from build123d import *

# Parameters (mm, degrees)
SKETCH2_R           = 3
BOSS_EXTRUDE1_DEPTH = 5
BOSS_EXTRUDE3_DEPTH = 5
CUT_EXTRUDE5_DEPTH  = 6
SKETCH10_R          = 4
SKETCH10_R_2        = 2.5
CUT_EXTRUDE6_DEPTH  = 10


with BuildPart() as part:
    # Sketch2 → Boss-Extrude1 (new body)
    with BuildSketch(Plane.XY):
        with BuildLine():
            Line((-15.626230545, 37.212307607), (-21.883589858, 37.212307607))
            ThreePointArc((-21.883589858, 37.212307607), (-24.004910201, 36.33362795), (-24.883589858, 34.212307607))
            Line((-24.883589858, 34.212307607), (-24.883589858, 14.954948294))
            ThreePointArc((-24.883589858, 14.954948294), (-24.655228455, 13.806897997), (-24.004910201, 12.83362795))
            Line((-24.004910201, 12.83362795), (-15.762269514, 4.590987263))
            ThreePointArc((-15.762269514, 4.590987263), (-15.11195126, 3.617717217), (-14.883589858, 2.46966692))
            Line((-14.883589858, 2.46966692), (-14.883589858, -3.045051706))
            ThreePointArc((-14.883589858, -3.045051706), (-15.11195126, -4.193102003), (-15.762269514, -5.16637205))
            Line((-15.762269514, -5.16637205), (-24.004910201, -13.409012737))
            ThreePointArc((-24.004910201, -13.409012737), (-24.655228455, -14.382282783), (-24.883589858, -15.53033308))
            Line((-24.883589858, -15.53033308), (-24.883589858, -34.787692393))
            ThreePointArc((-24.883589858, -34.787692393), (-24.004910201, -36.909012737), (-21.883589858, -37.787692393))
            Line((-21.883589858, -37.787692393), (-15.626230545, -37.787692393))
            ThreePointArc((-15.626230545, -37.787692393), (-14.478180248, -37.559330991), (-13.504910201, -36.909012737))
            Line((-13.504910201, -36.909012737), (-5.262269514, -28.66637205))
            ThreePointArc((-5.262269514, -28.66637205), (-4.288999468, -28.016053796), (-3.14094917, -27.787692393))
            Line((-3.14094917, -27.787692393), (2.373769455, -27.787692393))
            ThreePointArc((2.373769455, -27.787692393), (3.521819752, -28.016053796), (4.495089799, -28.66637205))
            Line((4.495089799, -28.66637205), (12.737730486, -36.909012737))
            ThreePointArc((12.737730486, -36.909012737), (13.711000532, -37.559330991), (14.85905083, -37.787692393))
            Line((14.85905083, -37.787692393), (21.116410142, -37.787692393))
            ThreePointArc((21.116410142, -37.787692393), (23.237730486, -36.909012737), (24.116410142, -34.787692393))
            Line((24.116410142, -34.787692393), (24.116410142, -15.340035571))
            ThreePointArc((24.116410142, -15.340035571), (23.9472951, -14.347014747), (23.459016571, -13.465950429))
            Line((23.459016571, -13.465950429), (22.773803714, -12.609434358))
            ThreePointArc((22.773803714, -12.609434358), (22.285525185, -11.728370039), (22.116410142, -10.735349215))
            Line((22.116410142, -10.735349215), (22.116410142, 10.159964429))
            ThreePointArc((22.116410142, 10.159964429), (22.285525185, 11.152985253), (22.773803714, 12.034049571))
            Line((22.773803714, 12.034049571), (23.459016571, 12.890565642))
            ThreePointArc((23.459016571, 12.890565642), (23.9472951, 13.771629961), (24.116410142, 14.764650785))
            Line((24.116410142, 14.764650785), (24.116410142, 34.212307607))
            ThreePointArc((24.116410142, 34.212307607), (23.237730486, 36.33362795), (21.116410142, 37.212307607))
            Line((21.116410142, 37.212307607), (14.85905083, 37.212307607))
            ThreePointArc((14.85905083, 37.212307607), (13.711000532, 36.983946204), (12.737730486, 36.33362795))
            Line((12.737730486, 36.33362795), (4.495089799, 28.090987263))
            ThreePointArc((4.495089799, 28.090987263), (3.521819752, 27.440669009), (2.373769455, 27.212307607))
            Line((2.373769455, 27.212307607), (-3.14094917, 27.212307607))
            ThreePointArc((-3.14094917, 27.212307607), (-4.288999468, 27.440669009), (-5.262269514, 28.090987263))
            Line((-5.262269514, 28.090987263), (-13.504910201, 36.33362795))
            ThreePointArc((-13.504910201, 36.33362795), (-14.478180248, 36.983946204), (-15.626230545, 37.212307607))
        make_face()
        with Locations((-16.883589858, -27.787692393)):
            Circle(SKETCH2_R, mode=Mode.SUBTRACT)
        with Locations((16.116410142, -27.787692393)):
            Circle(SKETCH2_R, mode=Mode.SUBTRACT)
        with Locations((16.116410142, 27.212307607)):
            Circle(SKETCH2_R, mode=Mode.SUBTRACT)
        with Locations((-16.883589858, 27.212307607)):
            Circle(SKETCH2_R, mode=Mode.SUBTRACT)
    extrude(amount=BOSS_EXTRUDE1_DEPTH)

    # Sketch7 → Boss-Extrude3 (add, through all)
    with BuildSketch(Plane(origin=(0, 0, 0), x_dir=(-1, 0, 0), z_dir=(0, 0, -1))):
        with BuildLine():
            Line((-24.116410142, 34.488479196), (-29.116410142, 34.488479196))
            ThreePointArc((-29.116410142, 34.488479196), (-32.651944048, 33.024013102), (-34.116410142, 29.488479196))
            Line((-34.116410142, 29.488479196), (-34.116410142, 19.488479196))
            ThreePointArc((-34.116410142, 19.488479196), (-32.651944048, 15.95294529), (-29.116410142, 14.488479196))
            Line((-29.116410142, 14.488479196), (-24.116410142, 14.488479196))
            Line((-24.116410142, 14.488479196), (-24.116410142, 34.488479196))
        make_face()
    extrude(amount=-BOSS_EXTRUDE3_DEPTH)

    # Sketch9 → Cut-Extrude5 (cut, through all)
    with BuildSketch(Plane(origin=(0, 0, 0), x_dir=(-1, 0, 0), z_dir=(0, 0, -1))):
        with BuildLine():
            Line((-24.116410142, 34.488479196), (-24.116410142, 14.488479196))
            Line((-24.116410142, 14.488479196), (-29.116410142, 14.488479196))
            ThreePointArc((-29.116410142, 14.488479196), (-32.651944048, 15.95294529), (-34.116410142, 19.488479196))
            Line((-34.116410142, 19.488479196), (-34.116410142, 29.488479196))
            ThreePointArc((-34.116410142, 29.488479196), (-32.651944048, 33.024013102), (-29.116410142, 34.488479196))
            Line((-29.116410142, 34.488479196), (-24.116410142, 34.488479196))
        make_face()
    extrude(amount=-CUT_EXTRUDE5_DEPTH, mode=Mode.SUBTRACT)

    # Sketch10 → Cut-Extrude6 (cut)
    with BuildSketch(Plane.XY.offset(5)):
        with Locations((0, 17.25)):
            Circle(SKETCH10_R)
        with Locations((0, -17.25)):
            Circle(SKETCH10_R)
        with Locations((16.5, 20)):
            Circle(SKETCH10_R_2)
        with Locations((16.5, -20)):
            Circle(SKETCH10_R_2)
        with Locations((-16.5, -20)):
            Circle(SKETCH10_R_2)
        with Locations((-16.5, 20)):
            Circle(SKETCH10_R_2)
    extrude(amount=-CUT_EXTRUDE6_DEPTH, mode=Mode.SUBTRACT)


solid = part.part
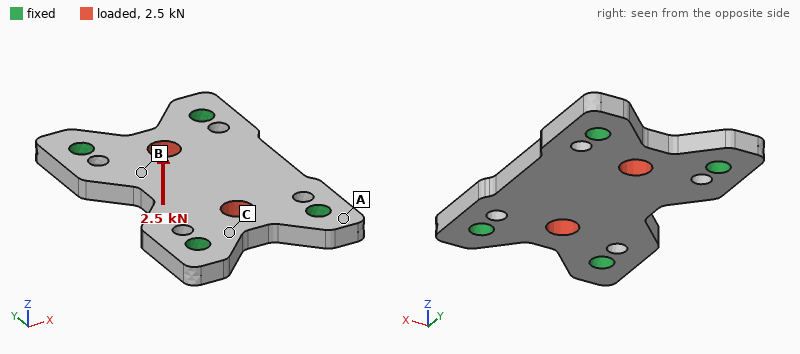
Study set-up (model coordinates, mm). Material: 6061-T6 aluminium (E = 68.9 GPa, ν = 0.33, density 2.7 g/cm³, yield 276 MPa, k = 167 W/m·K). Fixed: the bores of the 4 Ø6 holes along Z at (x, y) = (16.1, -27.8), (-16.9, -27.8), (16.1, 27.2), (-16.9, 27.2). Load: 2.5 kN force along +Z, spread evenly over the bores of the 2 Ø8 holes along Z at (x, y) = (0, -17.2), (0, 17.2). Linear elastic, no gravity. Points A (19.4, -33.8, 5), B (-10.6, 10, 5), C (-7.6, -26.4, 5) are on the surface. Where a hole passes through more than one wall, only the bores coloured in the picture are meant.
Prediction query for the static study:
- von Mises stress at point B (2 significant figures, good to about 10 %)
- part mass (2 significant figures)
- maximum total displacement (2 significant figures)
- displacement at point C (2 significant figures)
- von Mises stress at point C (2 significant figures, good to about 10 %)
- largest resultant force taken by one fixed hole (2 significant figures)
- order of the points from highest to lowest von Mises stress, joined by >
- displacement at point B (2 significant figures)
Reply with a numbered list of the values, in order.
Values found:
1. 23 MPa
2. 38 g
3. 46 µm
4. 11 µm
5. 35 MPa
6. 650 N
7. C > B > A
8. 33 µm
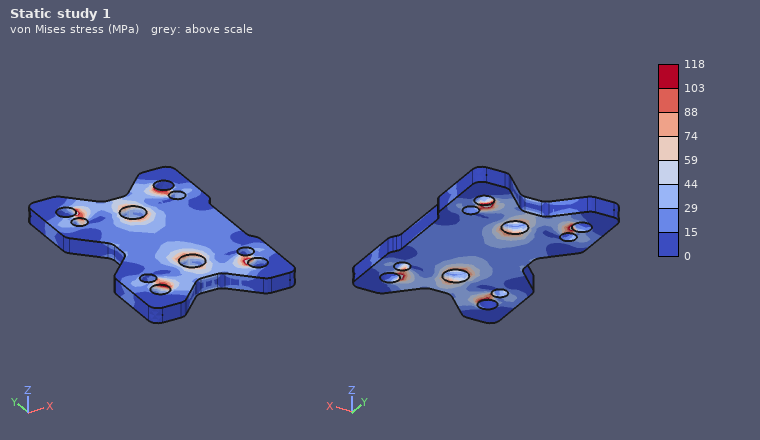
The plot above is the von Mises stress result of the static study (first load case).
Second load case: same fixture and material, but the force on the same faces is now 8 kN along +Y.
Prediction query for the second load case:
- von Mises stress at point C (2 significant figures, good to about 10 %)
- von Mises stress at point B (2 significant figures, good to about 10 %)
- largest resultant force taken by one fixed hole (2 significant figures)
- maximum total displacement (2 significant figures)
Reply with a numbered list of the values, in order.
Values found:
1. 26 MPa
2. 13 MPa
3. 2.3 kN
4. 14 µm
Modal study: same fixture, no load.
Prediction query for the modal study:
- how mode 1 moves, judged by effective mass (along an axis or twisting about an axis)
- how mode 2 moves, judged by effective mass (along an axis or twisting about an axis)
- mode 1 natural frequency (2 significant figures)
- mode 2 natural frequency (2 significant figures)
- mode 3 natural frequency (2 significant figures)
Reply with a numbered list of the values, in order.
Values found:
1. along Z
2. twisting about Y
3. 7900 Hz
4. 12 kHz
5. 19 kHz
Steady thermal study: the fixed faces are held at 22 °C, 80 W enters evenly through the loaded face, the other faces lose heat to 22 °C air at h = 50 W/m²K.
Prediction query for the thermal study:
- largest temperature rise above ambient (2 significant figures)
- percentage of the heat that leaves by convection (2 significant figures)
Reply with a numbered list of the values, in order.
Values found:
1. 24 K
2. 4.4 %
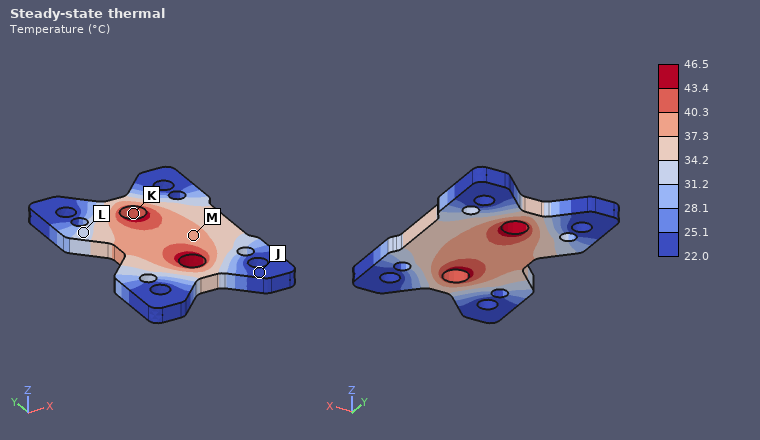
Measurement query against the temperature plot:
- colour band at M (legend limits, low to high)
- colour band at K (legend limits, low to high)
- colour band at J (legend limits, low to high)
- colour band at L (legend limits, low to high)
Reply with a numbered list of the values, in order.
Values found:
1. 37.3 to 40.3 °C
2. 40.3 to 43.4 °C
3. 22.0 to 25.1 °C
4. 31.2 to 34.2 °C
